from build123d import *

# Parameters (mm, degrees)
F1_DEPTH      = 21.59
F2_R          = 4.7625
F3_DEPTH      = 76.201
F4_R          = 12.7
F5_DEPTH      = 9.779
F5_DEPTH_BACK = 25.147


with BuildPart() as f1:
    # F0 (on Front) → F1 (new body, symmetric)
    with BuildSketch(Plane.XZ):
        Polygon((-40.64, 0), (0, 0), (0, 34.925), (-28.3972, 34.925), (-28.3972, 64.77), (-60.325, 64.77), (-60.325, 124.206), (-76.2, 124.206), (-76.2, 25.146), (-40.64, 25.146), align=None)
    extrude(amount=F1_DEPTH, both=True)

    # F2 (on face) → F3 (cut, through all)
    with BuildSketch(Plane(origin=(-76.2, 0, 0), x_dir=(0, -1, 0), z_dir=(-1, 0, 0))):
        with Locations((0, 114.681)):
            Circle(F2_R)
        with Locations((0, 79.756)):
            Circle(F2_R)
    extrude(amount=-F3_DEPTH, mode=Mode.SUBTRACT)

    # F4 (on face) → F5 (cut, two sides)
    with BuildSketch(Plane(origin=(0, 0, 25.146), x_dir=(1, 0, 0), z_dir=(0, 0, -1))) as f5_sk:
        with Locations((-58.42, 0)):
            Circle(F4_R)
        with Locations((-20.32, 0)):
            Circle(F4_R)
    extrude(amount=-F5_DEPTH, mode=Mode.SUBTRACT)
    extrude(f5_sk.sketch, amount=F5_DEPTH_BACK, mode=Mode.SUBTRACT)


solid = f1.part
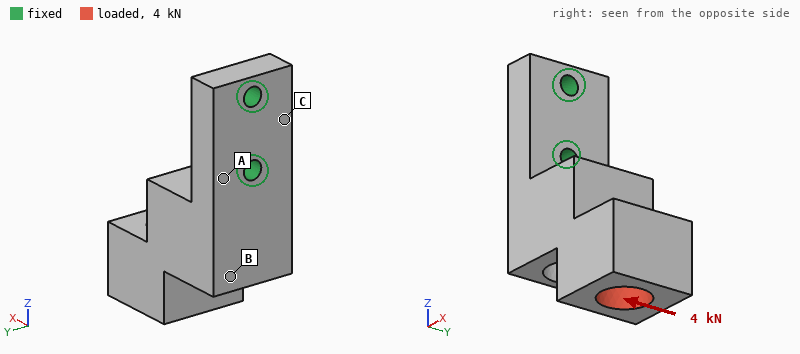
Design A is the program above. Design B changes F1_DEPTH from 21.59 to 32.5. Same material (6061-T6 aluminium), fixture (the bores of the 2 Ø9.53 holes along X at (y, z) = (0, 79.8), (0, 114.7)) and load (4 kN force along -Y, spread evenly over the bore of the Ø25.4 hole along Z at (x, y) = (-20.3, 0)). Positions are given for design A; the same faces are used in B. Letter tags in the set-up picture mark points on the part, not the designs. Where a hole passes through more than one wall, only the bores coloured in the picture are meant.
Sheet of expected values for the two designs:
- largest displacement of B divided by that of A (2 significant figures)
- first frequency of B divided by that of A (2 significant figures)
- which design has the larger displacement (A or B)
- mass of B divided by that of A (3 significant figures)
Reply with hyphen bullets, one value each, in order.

- 0.59
- 0.90
- A
- 1.59
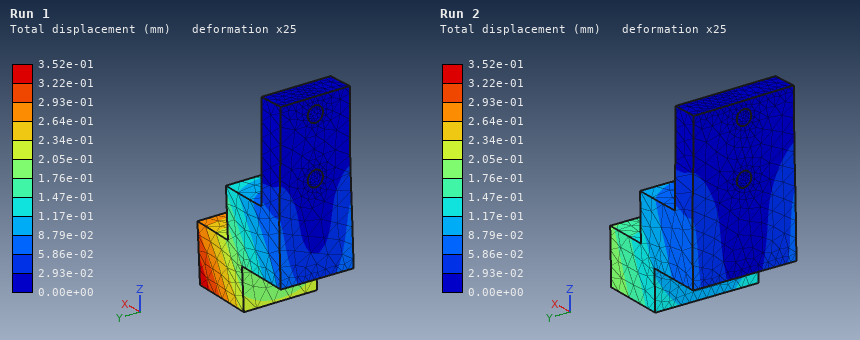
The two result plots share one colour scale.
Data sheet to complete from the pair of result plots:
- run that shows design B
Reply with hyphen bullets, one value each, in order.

- Run 2
